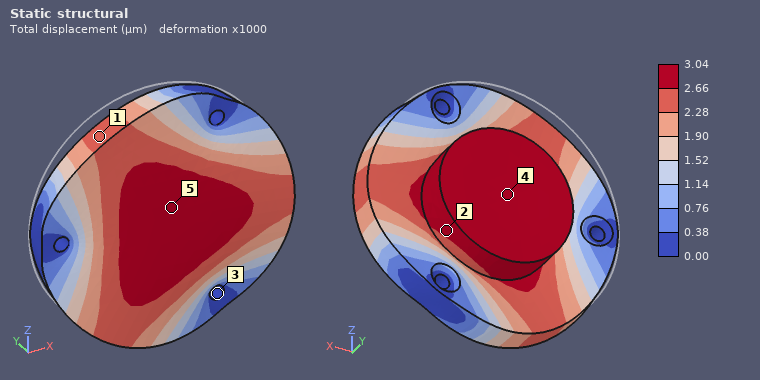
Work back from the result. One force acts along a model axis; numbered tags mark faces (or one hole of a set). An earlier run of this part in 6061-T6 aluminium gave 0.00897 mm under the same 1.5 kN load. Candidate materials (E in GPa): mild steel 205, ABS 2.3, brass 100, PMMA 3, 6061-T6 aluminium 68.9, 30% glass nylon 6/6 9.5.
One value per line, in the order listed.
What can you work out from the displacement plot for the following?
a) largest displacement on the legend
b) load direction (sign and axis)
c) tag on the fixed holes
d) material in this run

3.04 µm
-Y
3
mild steel
